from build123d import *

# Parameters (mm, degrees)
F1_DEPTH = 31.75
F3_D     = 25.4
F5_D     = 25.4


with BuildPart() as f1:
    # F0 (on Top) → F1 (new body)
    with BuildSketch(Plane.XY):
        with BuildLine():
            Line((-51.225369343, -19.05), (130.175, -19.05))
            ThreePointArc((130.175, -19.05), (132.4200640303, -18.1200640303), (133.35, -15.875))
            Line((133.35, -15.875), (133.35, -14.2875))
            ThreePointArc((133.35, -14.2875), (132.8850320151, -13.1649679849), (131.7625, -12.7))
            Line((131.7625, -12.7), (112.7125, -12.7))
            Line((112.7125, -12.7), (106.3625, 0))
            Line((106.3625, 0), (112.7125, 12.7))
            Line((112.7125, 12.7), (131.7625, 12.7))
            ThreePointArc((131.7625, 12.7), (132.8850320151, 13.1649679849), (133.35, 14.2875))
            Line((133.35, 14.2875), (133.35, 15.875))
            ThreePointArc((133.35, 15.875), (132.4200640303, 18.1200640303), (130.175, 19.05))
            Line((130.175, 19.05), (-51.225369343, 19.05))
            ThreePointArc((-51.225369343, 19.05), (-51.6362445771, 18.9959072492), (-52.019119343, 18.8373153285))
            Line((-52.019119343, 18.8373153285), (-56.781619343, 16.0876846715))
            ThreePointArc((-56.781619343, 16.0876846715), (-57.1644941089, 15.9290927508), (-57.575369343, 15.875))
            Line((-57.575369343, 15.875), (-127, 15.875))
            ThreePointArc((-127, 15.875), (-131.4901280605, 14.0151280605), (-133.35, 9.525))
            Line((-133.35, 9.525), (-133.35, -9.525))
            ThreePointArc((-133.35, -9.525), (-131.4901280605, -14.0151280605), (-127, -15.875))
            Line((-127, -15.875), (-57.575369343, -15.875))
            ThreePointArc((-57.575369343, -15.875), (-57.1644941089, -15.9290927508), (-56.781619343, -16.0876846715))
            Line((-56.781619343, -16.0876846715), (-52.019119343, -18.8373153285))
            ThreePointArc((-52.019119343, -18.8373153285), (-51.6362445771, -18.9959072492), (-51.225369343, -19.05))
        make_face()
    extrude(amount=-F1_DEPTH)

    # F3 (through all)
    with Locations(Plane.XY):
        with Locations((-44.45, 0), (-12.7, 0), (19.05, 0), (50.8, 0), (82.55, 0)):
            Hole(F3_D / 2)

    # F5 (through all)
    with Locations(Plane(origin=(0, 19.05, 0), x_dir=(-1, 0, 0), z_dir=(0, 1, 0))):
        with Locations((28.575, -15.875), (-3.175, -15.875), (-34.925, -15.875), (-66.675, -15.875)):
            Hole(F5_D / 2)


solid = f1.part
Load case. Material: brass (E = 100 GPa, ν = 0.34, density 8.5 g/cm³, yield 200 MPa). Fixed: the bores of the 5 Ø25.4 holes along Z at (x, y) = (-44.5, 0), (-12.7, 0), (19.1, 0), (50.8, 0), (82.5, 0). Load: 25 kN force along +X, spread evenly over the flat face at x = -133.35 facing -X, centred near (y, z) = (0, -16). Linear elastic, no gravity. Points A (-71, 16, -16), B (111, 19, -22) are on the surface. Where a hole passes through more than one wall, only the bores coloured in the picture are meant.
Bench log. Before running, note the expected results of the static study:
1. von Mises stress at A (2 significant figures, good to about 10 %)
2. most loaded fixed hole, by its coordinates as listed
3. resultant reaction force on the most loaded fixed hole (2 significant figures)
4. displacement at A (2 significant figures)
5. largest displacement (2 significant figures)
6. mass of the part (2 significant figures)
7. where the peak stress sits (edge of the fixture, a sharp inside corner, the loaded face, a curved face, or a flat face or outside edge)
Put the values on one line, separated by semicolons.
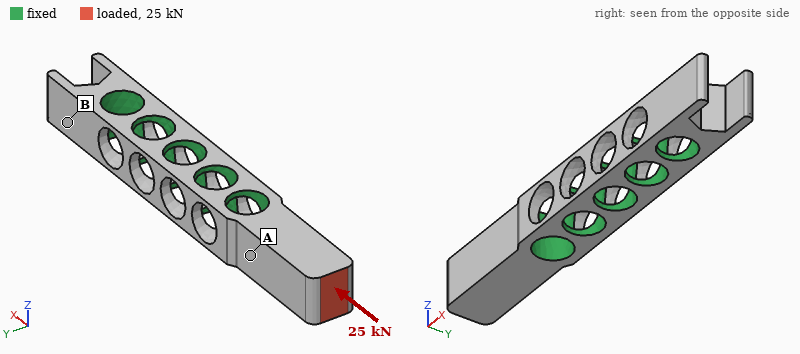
23 MPa; (-44.5, 0); 25 kN; 4.3 µm; 23 µm; 1.3 kg; the loaded face
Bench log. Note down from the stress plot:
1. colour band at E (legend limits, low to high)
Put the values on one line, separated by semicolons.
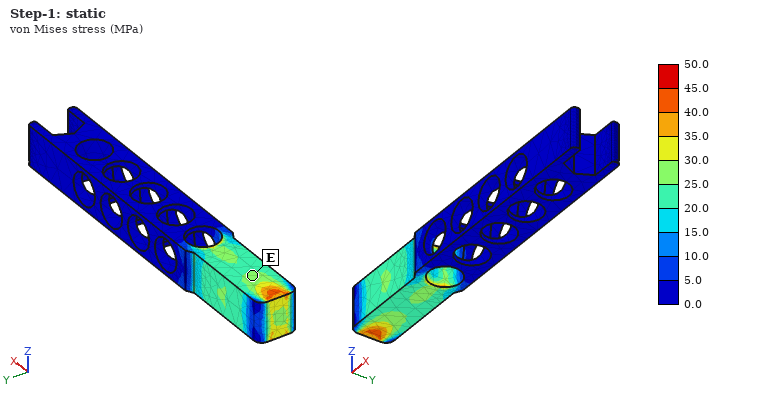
25.0 to 30.0 MPa
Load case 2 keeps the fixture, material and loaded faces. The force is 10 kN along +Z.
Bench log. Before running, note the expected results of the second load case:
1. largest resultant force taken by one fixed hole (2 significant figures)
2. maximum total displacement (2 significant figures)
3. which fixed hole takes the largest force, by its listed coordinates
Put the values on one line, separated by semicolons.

10.0 kN; 0.22 mm; (-44.5, 0)
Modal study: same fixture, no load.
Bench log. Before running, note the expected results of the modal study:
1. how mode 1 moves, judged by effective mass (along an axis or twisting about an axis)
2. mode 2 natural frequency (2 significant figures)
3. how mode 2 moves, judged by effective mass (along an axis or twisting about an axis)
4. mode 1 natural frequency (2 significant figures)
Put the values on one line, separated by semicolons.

along Y; 2600 Hz; along Z; 2400 Hz
